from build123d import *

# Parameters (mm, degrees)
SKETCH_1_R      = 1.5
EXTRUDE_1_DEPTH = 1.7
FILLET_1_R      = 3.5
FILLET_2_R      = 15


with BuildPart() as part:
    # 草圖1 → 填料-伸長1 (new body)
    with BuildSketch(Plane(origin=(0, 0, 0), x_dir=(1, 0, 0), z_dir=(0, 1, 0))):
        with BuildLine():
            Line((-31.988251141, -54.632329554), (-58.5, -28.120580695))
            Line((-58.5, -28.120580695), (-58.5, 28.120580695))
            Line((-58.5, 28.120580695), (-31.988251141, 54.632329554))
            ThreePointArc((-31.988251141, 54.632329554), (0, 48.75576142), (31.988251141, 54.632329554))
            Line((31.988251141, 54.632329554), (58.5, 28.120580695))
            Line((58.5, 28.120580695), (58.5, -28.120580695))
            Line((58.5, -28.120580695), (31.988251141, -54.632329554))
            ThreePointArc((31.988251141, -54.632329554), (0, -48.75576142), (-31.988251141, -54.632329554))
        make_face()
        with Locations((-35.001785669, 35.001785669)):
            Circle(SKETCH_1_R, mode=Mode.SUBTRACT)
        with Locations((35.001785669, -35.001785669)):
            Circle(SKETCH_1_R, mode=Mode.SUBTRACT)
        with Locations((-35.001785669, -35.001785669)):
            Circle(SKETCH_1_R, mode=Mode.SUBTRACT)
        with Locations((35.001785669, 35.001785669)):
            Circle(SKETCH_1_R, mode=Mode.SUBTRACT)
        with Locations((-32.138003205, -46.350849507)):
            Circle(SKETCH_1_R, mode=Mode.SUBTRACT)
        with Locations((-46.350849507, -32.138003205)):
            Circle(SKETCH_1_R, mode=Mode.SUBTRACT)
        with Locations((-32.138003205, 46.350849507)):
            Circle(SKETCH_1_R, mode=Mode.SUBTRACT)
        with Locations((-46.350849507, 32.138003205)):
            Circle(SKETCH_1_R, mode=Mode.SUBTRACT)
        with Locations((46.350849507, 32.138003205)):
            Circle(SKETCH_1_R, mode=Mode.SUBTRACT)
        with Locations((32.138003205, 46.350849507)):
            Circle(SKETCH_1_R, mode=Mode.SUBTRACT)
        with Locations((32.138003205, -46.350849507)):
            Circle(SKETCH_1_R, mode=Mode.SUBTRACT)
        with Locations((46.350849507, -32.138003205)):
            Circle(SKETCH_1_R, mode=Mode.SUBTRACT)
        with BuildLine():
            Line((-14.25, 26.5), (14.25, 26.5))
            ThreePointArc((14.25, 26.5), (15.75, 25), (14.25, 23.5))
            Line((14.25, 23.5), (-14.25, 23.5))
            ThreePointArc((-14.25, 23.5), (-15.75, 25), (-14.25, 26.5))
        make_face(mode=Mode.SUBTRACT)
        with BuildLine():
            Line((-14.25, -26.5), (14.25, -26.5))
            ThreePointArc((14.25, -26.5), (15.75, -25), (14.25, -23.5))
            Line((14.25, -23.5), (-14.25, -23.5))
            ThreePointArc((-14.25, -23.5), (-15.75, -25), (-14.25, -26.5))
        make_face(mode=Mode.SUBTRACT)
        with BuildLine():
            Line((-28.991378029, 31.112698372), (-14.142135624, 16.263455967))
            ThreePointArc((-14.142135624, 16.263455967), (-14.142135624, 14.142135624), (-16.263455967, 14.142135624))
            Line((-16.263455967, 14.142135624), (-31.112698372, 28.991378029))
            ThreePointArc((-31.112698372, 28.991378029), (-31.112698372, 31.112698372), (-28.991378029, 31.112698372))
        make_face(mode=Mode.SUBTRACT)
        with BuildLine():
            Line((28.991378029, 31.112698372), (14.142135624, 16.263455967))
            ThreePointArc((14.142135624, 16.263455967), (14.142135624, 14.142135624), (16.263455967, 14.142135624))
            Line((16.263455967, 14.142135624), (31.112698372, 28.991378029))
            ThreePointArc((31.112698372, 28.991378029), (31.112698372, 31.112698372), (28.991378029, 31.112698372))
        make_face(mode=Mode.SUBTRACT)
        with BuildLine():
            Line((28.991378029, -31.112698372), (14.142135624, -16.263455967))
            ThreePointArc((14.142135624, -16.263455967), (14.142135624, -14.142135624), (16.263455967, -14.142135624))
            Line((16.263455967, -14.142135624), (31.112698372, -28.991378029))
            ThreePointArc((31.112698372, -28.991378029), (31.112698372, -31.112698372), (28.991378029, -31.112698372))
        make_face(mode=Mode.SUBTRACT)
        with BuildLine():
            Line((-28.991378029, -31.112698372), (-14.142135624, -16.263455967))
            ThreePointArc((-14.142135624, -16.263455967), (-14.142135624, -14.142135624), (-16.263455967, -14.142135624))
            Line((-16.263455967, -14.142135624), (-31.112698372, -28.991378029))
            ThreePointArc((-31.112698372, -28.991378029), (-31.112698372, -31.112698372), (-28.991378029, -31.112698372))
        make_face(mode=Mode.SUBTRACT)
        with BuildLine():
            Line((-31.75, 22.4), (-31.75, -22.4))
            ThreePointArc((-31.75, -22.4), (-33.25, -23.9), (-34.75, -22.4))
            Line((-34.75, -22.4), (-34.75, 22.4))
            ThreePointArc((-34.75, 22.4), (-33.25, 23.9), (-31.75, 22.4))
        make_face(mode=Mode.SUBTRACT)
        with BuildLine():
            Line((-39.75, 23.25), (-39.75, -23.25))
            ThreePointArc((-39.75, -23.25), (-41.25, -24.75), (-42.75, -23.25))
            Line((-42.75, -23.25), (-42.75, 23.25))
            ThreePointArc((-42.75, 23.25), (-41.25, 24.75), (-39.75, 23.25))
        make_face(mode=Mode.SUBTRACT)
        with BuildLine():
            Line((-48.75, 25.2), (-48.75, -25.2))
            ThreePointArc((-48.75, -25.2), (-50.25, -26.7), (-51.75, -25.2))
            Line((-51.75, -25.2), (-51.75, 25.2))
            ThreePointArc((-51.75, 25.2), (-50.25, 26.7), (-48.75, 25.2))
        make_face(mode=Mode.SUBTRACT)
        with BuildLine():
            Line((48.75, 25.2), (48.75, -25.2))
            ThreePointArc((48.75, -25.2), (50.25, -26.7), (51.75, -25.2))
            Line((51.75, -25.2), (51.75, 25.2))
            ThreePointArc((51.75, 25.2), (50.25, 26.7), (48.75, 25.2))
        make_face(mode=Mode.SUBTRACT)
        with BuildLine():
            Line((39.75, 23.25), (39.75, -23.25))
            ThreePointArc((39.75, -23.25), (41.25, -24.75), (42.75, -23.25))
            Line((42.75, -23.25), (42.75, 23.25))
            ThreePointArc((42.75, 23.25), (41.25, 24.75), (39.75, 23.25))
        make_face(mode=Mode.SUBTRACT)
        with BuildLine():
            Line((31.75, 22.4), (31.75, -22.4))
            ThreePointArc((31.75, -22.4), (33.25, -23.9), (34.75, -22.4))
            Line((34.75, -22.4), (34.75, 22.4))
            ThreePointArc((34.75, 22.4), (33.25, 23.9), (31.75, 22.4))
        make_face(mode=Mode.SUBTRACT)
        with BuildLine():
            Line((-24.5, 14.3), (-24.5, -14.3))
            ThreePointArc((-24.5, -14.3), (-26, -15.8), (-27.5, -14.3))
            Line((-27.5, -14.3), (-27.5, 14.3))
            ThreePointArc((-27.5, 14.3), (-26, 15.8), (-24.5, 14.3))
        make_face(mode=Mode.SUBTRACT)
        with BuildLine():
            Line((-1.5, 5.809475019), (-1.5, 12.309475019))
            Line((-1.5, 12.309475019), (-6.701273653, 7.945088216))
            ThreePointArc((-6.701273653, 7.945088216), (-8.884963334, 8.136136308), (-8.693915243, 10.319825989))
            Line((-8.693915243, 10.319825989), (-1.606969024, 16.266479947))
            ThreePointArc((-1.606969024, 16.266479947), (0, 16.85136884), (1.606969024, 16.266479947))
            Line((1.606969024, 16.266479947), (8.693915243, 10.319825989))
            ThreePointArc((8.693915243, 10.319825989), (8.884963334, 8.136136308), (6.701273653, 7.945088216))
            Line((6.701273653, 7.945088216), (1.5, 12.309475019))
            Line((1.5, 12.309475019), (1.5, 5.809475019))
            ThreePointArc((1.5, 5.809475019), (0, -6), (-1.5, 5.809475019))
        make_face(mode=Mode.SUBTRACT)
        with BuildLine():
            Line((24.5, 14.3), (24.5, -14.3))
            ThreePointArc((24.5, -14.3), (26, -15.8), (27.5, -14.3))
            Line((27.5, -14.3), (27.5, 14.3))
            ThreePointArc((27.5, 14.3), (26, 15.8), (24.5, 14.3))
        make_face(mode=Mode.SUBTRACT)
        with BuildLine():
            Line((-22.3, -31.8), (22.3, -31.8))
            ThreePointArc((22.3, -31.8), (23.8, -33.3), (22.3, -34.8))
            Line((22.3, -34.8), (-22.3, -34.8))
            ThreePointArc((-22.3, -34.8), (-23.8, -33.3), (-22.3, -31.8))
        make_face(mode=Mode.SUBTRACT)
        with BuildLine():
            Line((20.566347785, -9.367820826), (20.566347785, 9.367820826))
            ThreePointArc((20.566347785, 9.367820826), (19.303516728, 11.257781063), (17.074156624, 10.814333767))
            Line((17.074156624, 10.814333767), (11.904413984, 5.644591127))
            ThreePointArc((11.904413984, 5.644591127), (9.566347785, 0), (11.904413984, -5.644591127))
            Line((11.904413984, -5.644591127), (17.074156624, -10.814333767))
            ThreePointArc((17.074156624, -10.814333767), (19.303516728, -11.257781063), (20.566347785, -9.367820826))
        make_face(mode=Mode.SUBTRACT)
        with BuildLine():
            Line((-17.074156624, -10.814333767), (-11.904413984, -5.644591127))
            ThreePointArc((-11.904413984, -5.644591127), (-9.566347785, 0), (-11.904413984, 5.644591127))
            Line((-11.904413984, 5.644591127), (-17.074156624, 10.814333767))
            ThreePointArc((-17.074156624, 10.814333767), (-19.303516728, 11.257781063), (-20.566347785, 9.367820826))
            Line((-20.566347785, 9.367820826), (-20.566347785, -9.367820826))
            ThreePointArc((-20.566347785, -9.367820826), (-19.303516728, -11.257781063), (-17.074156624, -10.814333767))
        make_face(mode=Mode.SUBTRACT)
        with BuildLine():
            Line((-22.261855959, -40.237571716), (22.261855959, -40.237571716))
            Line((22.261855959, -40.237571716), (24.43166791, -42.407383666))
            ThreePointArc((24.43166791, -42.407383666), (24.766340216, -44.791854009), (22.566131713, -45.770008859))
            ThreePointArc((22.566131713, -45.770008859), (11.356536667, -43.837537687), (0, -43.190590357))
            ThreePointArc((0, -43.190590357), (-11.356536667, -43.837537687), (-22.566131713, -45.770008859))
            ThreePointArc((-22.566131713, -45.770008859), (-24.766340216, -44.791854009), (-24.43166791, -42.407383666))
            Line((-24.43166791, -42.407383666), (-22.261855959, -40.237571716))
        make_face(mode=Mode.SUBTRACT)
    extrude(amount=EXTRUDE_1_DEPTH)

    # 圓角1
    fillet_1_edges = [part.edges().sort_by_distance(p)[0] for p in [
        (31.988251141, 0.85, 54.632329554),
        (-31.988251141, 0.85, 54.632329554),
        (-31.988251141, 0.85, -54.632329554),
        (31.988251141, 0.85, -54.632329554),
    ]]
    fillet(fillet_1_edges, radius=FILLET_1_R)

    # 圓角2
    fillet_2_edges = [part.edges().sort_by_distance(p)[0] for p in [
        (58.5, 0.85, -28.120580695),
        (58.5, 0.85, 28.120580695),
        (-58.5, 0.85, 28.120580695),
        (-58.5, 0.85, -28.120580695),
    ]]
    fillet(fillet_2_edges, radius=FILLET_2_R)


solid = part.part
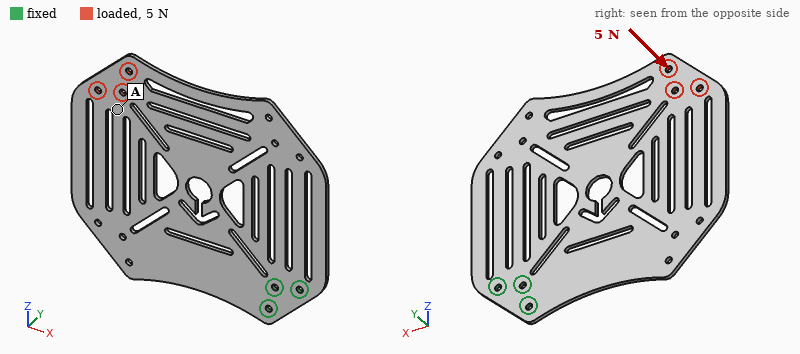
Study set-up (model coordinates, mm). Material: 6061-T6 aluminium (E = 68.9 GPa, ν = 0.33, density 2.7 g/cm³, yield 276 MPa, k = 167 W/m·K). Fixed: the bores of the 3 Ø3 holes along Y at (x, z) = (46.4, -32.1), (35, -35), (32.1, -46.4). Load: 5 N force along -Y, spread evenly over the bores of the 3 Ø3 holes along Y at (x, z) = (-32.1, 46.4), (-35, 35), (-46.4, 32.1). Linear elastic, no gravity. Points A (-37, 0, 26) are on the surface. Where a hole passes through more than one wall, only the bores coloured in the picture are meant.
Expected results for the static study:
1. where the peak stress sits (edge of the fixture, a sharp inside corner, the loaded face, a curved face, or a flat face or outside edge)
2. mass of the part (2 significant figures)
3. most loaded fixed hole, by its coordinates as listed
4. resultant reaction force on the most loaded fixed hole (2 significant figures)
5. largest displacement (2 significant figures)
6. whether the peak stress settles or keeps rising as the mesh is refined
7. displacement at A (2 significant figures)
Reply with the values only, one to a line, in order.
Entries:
edge of the fixture
38 g
(35, -35)
22 N
1.7 mm
keeps rising
1.3 mm
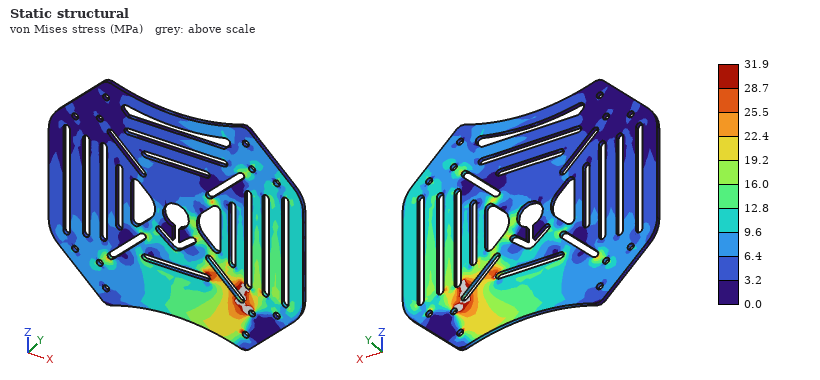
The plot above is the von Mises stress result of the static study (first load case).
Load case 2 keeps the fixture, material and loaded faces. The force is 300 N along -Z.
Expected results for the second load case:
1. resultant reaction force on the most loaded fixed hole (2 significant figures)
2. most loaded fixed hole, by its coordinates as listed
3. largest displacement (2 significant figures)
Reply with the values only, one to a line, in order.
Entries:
1.1 kN
(32.1, -46.4)
0.29 mm
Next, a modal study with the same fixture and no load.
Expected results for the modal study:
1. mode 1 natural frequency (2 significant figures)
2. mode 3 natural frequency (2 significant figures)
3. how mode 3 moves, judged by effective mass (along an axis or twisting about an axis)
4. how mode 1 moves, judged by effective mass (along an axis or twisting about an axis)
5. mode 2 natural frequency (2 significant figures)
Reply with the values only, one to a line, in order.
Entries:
96 Hz
410 Hz
along Y
along Y
200 Hz
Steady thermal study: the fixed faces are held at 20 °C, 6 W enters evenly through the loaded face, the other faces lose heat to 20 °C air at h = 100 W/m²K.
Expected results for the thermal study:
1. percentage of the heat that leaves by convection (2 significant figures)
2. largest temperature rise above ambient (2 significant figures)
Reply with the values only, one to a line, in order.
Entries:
97 %
16 K
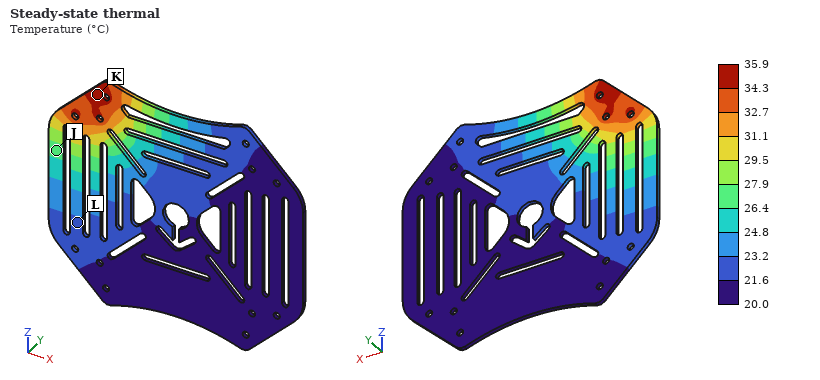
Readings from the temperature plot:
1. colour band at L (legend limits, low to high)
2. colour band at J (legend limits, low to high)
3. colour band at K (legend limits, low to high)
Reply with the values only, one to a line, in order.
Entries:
21.6 to 23.2 °C
26.4 to 27.9 °C
34.3 to 35.9 °C
